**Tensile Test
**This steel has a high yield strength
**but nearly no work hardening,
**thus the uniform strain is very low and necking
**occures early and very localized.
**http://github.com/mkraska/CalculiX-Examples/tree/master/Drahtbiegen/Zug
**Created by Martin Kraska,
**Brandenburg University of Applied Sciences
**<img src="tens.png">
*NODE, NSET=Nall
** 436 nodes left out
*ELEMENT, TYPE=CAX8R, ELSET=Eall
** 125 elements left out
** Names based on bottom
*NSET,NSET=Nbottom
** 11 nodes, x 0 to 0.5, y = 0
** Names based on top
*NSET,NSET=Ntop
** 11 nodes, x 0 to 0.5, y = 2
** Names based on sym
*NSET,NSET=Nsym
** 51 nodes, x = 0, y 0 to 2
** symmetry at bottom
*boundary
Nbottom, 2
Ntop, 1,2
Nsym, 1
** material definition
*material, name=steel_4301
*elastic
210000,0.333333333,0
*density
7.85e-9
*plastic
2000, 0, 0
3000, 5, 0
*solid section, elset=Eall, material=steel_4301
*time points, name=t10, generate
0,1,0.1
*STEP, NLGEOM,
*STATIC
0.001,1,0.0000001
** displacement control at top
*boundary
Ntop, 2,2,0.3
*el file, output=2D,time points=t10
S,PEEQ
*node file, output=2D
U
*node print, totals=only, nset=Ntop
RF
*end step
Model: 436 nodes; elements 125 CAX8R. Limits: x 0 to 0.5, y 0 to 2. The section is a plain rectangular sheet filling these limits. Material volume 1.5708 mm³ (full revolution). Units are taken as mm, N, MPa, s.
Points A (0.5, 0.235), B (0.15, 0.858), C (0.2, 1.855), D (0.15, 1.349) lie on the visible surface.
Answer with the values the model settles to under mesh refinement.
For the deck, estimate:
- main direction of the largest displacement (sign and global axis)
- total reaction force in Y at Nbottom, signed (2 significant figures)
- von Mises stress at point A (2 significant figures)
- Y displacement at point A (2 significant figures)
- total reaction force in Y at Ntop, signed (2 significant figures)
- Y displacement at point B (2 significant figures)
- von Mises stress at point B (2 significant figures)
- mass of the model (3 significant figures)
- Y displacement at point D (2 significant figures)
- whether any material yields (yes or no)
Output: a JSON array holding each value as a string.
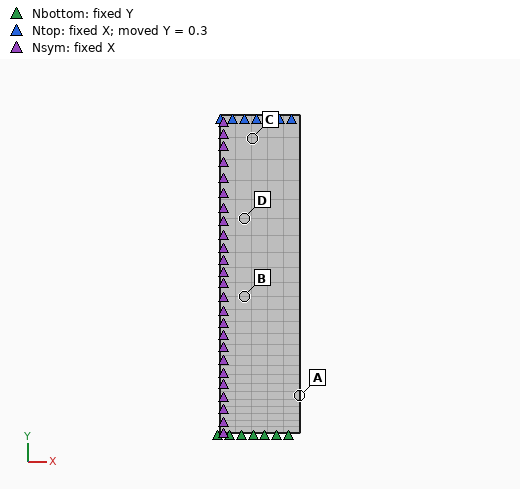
["+Y", "-600 N", "2000 MPa", "0.22 mm", "600 N", "0.29 mm", "450 MPa", "1.23e-05 kg", "0.30 mm", "yes"]
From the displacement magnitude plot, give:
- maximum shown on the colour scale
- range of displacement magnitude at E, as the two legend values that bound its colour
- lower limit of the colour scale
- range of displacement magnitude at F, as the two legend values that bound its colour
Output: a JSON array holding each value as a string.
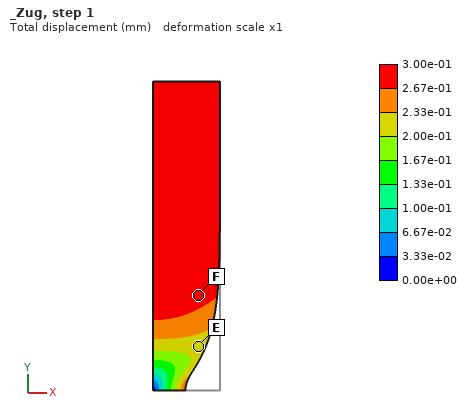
["3.00e-01 mm", "2.00e-01 to 2.33e-01 mm", "0.00e+00 mm", "2.67e-01 to 3.00e-01 mm"]
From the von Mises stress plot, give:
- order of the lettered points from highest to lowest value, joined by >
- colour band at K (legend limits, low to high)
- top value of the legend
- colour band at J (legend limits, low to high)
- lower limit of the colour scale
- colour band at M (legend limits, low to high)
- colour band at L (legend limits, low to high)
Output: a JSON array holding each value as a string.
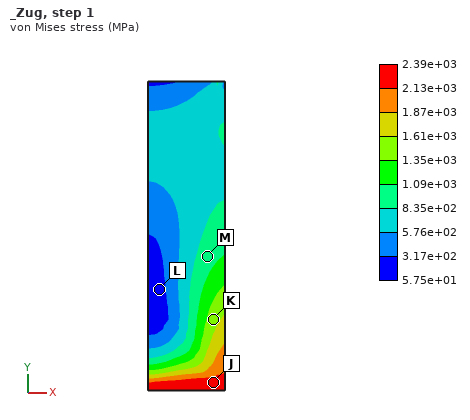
["J > K > M > L", "1.35e+03 to 1.61e+03 MPa", "2.39e+03 MPa", "2.13e+03 to 2.39e+03 MPa", "5.75e+01 MPa", "8.35e+02 to 1.09e+03 MPa", "5.75e+01 to 3.17e+02 MPa"]
